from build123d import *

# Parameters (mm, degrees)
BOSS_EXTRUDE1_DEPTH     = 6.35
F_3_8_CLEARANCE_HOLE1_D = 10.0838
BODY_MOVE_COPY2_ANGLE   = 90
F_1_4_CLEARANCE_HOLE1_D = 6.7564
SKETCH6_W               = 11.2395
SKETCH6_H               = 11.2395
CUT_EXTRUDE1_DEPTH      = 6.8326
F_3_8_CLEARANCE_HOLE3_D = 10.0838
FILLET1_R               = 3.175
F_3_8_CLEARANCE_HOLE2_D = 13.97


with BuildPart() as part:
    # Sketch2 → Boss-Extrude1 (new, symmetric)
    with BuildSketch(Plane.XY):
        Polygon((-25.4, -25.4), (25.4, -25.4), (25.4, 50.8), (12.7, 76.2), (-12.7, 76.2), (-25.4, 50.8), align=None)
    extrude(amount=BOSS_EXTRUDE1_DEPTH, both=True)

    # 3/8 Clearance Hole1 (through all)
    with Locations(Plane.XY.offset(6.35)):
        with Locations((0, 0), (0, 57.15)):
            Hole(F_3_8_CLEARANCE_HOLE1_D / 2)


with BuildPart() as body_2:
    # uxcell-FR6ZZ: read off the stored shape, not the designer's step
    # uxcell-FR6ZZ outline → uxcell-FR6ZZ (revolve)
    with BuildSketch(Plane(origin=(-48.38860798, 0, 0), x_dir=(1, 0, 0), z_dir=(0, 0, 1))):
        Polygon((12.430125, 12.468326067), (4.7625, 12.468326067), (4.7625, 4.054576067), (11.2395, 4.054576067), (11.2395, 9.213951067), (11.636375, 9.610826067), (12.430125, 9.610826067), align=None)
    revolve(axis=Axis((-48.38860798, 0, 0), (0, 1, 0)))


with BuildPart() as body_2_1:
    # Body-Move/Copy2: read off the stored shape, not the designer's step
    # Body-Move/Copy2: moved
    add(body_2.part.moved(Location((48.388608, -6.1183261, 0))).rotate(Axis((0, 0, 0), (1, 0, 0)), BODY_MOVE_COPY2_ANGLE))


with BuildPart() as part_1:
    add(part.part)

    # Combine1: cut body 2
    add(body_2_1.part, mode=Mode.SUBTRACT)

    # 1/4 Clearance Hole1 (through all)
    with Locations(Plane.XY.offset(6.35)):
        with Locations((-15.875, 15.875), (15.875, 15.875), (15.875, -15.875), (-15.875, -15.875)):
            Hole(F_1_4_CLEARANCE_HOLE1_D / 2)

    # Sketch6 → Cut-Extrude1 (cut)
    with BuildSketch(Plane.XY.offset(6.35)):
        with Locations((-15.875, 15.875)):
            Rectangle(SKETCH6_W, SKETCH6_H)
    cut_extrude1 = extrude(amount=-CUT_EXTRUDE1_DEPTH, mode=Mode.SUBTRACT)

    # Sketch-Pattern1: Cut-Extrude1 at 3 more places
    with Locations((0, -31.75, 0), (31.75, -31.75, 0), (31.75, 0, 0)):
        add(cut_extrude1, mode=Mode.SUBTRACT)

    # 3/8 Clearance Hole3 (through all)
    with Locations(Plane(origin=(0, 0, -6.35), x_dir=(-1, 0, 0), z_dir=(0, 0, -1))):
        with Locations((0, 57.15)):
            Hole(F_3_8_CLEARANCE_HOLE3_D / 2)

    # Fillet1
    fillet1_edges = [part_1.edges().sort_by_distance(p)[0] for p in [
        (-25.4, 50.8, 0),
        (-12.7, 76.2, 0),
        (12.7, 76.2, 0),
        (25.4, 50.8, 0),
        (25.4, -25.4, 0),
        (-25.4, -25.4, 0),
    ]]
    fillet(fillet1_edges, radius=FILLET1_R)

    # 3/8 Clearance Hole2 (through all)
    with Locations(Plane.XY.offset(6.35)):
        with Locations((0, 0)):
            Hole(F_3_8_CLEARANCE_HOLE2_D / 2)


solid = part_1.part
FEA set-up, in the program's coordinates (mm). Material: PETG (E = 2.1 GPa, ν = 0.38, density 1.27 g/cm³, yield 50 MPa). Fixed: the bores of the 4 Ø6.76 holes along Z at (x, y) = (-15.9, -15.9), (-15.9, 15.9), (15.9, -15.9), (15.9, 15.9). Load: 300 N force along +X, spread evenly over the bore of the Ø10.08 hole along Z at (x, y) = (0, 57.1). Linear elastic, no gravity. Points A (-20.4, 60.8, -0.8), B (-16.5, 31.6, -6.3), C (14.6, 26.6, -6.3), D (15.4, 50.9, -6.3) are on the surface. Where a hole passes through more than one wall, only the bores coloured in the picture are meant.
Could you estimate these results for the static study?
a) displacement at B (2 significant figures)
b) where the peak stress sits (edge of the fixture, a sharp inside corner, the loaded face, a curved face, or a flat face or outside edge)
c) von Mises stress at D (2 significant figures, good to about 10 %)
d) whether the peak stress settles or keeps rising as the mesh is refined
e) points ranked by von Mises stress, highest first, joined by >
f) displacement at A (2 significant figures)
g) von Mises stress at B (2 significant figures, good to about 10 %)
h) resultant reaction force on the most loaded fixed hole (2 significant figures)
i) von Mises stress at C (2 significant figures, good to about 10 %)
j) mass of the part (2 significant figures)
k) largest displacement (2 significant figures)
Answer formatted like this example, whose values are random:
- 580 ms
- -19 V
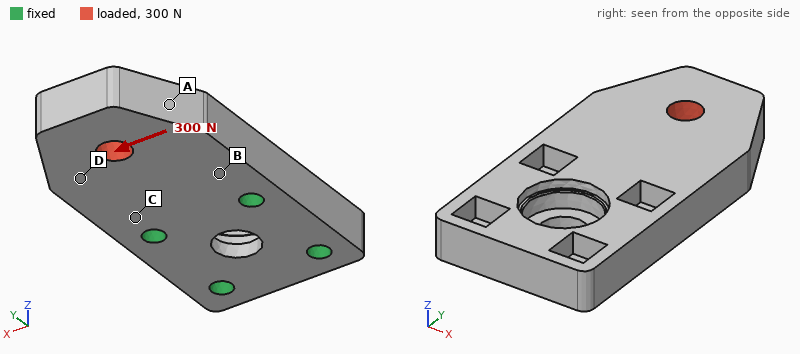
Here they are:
- 0.029 mm
- edge of the fixture
- 0.89 MPa
- keeps rising
- C > B > D > A
- 0.083 mm
- 1.7 MPa
- 330 N
- 2.3 MPa
- 66 g
- 0.10 mm
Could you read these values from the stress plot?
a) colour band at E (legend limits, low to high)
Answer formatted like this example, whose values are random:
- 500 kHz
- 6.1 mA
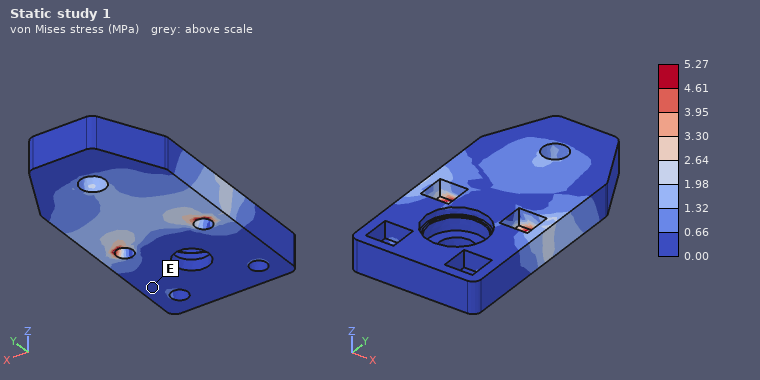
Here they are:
- 0.00 to 0.66 MPa
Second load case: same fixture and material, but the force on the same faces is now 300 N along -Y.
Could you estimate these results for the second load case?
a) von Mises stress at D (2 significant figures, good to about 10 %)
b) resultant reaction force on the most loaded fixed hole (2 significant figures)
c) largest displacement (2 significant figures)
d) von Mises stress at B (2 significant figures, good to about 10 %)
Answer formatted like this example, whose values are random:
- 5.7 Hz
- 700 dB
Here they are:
- 0.42 MPa
- 120 N
- 63 µm
- 0.57 MPa
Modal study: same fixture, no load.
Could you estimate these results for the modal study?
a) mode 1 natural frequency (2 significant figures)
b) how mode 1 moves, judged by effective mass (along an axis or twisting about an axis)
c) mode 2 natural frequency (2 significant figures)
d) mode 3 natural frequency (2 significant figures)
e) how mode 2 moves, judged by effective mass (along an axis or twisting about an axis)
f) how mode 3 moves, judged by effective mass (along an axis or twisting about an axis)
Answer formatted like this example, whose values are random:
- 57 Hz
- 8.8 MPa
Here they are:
- 620 Hz
- along Z
- 1900 Hz
- 2100 Hz
- along X
- along X
